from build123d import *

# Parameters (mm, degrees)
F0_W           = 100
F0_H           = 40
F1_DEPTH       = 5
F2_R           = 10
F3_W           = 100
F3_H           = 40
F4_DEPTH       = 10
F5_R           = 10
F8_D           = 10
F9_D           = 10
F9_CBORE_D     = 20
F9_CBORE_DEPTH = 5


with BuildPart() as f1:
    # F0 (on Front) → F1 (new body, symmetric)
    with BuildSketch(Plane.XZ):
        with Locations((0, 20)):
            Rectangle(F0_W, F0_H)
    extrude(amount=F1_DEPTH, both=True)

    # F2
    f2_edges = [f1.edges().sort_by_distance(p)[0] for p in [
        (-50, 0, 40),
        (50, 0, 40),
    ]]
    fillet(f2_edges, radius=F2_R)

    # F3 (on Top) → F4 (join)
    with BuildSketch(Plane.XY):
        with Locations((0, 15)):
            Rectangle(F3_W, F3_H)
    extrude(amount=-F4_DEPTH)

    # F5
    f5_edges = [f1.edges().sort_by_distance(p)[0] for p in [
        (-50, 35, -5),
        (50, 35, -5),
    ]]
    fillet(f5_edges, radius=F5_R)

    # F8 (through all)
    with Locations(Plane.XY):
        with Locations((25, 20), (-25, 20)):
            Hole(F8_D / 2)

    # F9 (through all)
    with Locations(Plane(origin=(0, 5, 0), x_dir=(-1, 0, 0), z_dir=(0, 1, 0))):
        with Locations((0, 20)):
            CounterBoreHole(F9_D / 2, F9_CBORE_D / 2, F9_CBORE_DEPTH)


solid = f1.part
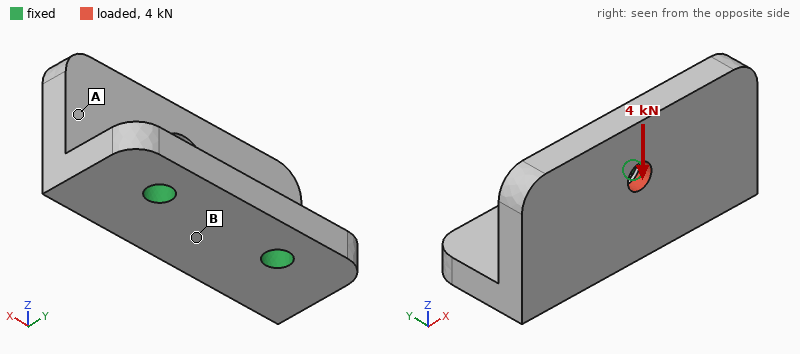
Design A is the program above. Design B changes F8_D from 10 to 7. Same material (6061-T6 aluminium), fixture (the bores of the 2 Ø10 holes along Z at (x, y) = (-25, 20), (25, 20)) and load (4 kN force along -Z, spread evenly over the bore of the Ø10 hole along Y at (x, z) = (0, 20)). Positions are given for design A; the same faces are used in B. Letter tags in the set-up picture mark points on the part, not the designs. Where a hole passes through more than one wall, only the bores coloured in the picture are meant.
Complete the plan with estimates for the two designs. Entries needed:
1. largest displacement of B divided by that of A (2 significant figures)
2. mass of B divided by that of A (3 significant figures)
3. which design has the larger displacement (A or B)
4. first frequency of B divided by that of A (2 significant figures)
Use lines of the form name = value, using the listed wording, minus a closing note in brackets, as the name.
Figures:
largest displacement of B divided by that of A = 1.2
mass of B divided by that of A = 1.01
which design has the larger displacement = B
first frequency of B divided by that of A = 0.93
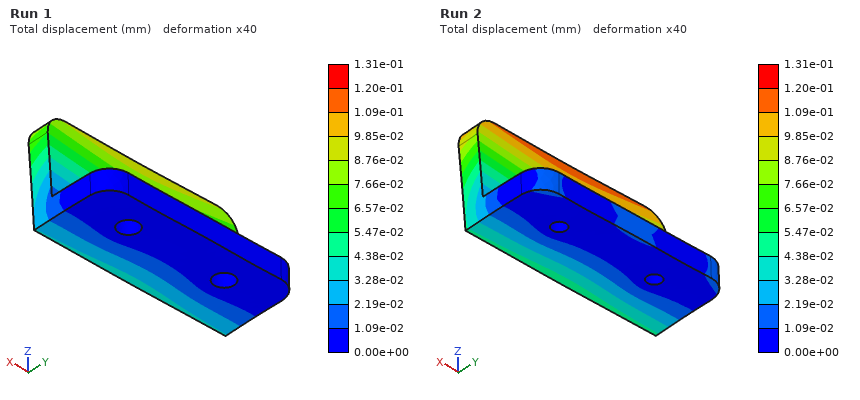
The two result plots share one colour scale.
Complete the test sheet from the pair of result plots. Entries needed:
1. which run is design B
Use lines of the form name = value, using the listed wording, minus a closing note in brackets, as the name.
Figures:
which run is design B = Run 2
